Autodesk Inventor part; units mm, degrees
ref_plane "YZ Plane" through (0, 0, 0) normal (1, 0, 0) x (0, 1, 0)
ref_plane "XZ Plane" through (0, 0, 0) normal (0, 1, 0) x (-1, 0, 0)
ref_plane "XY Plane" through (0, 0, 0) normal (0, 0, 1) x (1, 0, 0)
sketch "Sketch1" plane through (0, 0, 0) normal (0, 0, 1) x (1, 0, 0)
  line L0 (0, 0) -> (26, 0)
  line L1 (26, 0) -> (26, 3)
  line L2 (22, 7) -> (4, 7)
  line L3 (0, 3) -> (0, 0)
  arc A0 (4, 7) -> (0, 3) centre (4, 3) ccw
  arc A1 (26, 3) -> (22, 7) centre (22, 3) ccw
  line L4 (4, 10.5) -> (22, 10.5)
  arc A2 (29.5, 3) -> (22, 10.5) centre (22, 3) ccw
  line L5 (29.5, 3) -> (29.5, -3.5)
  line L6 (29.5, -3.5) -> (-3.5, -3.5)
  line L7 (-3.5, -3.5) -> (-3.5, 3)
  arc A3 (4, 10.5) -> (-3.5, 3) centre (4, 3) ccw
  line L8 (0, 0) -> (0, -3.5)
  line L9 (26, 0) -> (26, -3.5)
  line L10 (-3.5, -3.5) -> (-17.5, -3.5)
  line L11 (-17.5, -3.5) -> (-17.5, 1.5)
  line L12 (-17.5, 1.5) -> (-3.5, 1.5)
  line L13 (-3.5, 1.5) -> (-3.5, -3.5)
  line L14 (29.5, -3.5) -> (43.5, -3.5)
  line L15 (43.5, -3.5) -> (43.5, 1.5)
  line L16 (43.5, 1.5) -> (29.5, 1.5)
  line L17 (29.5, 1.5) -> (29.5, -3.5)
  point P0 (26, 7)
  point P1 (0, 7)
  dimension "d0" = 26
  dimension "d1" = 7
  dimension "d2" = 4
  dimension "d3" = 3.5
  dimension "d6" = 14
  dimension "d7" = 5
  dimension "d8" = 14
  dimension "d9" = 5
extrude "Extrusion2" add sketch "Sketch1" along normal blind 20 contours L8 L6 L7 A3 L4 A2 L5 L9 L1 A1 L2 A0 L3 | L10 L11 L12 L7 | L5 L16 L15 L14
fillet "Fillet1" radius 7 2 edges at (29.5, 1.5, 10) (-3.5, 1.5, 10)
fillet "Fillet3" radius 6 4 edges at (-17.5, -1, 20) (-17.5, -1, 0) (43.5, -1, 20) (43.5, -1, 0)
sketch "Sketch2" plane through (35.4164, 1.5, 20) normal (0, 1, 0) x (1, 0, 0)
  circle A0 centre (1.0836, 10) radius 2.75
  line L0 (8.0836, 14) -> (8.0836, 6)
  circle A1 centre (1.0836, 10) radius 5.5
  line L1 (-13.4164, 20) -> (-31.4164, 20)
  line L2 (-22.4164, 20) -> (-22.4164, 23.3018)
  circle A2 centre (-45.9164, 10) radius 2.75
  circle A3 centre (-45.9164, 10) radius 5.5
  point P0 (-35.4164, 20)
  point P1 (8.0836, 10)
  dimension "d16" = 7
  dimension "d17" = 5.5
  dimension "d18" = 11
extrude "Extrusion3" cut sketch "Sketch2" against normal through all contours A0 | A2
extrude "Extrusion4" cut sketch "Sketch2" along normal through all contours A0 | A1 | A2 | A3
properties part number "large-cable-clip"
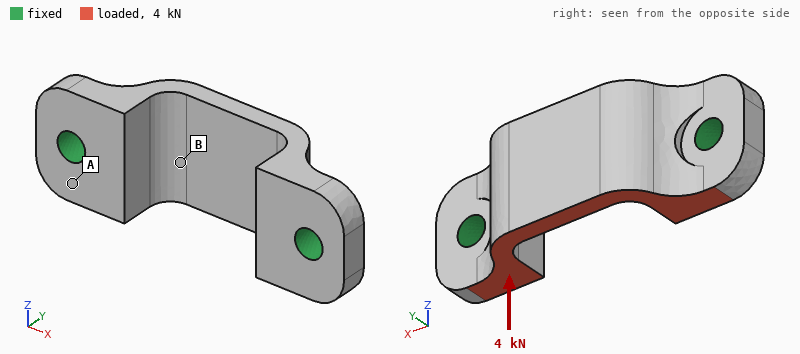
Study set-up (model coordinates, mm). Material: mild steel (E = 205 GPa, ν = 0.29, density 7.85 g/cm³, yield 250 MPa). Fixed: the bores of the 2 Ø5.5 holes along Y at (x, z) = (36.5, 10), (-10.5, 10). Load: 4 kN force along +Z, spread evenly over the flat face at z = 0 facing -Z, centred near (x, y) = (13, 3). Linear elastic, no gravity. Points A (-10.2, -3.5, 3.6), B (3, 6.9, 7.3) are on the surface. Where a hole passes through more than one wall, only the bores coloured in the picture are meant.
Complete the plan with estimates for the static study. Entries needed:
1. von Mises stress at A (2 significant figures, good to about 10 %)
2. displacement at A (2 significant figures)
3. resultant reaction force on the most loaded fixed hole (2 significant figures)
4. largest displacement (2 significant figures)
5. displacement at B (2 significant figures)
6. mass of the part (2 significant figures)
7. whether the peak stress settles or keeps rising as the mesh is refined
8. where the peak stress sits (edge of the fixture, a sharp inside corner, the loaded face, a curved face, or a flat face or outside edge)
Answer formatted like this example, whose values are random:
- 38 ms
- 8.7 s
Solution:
- 51 MPa
- 3.2 µm
- 2.0 kN
- 20 µm
- 12 µm
- 48 g
- keeps rising
- edge of the fixture
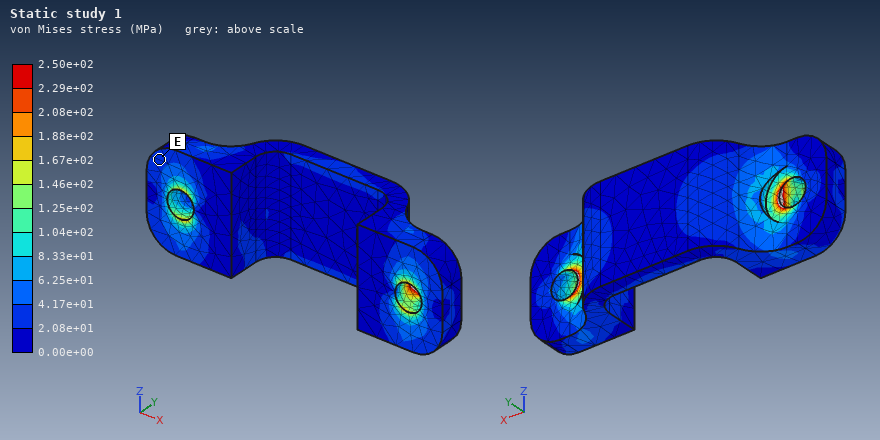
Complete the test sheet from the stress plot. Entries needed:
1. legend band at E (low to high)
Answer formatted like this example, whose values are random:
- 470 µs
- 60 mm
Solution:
- 2.08e+01 to 4.17e+01 MPa
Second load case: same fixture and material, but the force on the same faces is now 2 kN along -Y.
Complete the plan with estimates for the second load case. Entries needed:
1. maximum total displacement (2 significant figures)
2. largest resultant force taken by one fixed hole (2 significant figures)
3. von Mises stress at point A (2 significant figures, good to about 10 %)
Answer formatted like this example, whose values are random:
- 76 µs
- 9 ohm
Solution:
- 23 µm
- 1.1 kN
- 53 MPa
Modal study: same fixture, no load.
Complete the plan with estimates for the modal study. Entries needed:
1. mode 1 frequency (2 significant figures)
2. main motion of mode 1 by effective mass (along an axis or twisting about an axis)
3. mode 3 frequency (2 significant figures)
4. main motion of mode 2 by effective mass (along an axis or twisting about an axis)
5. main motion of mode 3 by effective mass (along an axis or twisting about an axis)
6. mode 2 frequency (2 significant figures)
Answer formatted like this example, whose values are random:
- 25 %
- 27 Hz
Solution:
- 13 kHz
- along Z
- 19 kHz
- along X
- along Y
- 16 kHz
